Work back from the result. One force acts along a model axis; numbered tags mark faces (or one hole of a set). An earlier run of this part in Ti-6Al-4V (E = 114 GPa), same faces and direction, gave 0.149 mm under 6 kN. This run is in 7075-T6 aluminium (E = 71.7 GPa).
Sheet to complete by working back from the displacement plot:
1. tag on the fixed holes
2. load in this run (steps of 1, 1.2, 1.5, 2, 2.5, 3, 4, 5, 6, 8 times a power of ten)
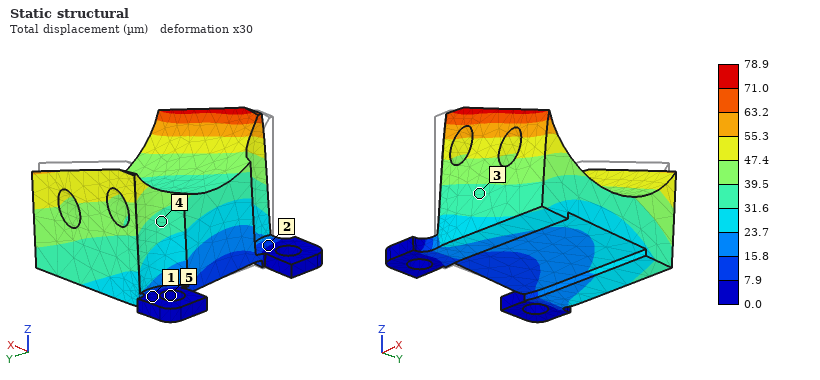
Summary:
5
2 kN
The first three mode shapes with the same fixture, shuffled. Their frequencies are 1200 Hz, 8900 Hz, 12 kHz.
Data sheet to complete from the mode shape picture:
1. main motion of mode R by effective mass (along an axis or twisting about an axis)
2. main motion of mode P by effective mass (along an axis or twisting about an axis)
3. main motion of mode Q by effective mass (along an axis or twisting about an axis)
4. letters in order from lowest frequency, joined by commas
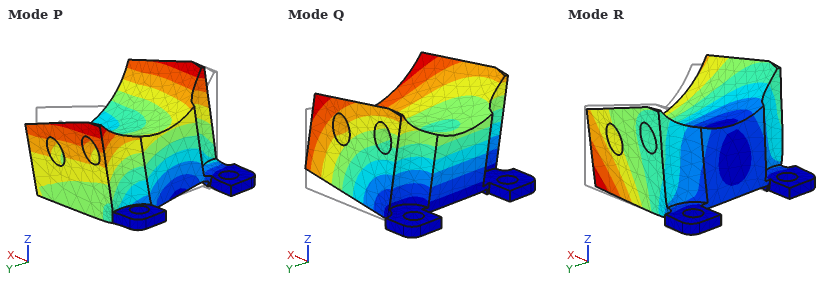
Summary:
along Y
along Y
along Z
Q, P, R
